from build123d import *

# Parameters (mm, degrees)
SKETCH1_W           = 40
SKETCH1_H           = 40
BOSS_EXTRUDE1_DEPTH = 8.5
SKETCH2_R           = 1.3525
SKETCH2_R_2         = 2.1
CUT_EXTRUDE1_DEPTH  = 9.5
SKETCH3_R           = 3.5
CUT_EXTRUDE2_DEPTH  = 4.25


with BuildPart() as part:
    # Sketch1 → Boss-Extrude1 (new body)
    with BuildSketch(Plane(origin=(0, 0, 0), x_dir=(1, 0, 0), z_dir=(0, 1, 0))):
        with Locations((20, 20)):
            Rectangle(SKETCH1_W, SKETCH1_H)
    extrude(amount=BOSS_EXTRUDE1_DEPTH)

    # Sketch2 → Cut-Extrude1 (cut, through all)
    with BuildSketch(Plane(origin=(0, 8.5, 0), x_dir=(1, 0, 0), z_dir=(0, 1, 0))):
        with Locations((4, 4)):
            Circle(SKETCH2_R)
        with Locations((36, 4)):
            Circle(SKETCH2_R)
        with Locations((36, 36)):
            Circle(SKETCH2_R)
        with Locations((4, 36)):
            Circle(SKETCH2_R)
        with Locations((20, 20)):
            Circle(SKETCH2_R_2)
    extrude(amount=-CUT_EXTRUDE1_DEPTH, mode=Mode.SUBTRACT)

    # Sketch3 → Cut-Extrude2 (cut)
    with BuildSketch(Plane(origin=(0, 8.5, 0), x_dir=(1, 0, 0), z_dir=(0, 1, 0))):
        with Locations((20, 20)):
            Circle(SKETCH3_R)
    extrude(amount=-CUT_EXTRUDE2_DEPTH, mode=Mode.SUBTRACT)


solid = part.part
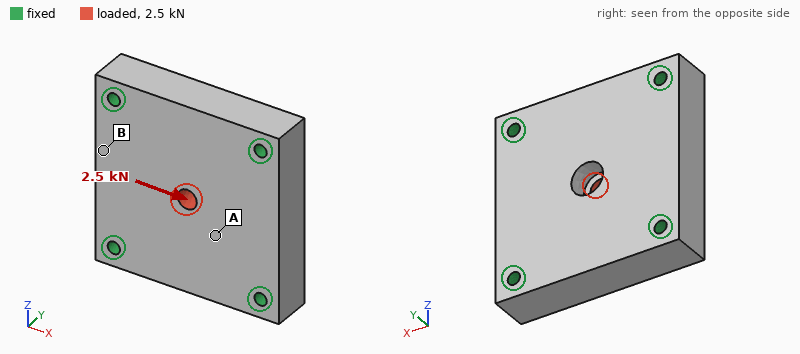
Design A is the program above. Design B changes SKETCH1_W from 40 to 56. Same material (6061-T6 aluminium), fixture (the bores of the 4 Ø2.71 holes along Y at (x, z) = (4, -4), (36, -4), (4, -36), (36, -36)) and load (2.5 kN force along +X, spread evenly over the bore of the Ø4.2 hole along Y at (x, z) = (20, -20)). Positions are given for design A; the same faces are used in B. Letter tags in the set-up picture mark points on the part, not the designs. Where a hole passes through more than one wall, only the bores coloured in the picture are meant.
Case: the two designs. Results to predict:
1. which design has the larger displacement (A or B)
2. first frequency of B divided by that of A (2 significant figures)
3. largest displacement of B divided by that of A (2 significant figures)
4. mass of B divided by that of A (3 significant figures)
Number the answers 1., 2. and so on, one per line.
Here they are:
1. A
2. 1.0
3. 0.92
4. 1.41
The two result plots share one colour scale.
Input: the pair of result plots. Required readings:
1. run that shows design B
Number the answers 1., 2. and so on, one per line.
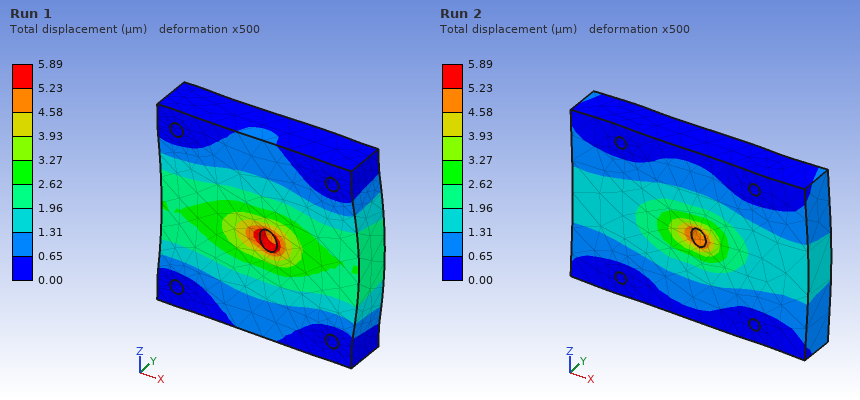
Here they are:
1. Run 2
